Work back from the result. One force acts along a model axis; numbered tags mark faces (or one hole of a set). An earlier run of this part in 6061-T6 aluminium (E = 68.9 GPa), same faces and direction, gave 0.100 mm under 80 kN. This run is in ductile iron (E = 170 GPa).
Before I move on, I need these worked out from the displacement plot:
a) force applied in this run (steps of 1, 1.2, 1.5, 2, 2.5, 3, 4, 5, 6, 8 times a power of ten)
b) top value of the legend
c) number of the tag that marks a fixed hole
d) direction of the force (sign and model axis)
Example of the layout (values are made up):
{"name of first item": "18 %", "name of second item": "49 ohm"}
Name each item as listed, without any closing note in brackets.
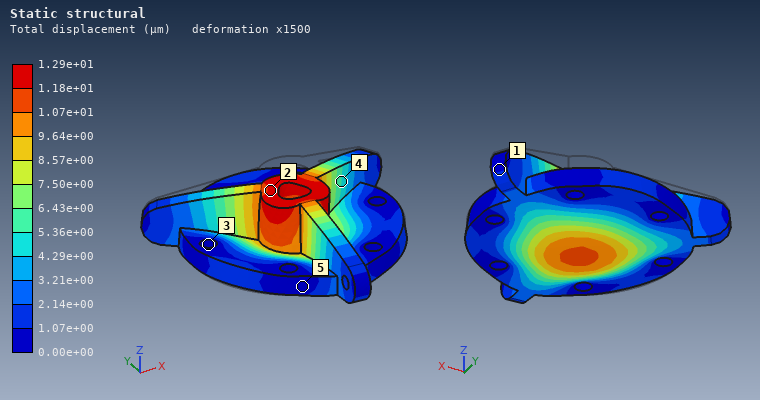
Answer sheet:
{"force applied in this run": "25 kN", "top value of the legend": "1.29e+01 µm", "number of the tag that marks a fixed hole": "3", "direction of the force": "-Z"}
